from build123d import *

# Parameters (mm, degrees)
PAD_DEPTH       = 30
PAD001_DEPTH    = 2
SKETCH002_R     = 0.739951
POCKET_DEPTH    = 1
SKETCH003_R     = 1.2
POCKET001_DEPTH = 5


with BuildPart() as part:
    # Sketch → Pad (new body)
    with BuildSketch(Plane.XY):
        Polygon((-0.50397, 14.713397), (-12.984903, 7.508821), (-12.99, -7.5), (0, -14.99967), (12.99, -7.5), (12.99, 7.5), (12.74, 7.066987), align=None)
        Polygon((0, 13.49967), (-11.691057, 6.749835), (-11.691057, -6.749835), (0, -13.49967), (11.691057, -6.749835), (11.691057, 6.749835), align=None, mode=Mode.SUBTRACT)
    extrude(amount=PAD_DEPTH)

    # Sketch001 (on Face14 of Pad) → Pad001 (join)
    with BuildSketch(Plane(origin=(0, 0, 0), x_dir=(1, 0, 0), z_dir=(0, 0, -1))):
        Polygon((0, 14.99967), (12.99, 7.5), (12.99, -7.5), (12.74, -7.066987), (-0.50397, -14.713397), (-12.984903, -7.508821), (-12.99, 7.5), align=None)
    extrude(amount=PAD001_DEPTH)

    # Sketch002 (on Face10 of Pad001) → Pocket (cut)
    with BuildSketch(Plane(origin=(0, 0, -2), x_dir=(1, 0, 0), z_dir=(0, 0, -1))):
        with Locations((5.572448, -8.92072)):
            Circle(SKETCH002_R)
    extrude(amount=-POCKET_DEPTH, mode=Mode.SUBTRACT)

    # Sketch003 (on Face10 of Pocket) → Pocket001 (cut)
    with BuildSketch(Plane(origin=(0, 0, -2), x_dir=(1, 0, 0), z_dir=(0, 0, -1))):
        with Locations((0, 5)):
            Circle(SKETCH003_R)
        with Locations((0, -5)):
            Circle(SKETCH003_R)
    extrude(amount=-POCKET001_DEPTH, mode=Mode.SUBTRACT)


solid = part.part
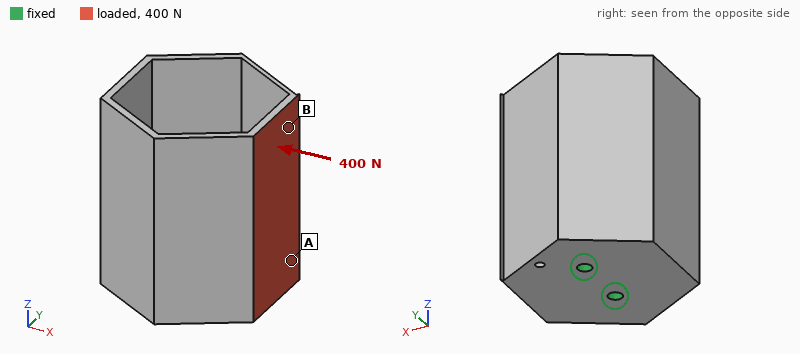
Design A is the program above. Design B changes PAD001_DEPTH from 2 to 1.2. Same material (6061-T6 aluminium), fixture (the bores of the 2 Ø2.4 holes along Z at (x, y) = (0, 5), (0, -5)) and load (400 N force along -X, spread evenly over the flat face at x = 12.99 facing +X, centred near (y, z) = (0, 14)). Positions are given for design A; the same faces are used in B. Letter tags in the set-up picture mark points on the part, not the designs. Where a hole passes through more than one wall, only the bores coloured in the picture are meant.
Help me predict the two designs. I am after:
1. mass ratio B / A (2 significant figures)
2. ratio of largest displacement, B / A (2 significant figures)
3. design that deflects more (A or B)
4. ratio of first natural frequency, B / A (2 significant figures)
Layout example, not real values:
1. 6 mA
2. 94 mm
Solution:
1. 0.89
2. 3.0
3. B
4. 0.54
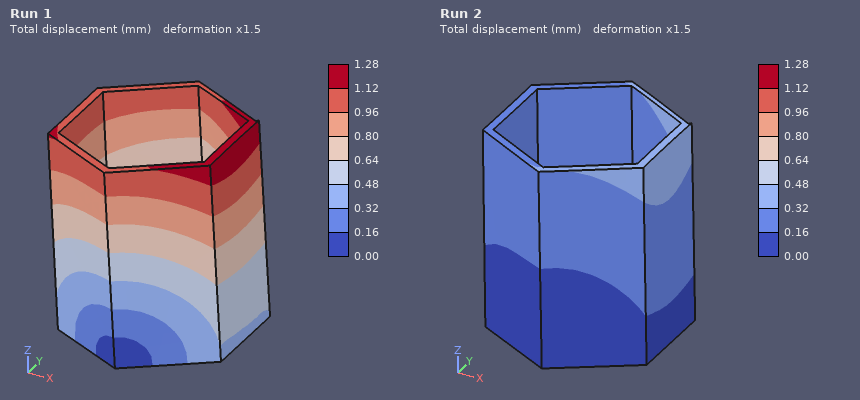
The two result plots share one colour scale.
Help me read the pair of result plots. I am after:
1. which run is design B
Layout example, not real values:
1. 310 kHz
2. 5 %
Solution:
1. Run 1
